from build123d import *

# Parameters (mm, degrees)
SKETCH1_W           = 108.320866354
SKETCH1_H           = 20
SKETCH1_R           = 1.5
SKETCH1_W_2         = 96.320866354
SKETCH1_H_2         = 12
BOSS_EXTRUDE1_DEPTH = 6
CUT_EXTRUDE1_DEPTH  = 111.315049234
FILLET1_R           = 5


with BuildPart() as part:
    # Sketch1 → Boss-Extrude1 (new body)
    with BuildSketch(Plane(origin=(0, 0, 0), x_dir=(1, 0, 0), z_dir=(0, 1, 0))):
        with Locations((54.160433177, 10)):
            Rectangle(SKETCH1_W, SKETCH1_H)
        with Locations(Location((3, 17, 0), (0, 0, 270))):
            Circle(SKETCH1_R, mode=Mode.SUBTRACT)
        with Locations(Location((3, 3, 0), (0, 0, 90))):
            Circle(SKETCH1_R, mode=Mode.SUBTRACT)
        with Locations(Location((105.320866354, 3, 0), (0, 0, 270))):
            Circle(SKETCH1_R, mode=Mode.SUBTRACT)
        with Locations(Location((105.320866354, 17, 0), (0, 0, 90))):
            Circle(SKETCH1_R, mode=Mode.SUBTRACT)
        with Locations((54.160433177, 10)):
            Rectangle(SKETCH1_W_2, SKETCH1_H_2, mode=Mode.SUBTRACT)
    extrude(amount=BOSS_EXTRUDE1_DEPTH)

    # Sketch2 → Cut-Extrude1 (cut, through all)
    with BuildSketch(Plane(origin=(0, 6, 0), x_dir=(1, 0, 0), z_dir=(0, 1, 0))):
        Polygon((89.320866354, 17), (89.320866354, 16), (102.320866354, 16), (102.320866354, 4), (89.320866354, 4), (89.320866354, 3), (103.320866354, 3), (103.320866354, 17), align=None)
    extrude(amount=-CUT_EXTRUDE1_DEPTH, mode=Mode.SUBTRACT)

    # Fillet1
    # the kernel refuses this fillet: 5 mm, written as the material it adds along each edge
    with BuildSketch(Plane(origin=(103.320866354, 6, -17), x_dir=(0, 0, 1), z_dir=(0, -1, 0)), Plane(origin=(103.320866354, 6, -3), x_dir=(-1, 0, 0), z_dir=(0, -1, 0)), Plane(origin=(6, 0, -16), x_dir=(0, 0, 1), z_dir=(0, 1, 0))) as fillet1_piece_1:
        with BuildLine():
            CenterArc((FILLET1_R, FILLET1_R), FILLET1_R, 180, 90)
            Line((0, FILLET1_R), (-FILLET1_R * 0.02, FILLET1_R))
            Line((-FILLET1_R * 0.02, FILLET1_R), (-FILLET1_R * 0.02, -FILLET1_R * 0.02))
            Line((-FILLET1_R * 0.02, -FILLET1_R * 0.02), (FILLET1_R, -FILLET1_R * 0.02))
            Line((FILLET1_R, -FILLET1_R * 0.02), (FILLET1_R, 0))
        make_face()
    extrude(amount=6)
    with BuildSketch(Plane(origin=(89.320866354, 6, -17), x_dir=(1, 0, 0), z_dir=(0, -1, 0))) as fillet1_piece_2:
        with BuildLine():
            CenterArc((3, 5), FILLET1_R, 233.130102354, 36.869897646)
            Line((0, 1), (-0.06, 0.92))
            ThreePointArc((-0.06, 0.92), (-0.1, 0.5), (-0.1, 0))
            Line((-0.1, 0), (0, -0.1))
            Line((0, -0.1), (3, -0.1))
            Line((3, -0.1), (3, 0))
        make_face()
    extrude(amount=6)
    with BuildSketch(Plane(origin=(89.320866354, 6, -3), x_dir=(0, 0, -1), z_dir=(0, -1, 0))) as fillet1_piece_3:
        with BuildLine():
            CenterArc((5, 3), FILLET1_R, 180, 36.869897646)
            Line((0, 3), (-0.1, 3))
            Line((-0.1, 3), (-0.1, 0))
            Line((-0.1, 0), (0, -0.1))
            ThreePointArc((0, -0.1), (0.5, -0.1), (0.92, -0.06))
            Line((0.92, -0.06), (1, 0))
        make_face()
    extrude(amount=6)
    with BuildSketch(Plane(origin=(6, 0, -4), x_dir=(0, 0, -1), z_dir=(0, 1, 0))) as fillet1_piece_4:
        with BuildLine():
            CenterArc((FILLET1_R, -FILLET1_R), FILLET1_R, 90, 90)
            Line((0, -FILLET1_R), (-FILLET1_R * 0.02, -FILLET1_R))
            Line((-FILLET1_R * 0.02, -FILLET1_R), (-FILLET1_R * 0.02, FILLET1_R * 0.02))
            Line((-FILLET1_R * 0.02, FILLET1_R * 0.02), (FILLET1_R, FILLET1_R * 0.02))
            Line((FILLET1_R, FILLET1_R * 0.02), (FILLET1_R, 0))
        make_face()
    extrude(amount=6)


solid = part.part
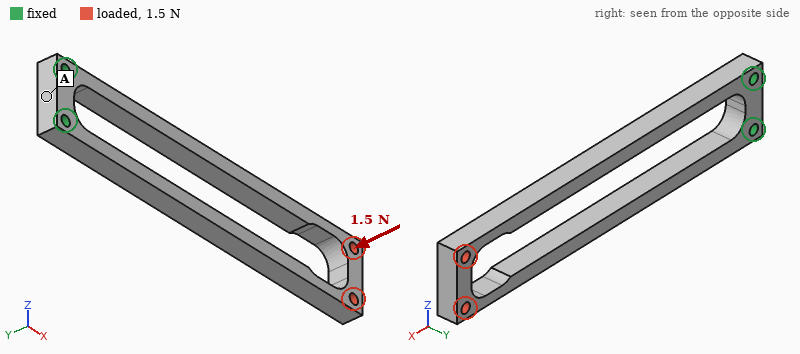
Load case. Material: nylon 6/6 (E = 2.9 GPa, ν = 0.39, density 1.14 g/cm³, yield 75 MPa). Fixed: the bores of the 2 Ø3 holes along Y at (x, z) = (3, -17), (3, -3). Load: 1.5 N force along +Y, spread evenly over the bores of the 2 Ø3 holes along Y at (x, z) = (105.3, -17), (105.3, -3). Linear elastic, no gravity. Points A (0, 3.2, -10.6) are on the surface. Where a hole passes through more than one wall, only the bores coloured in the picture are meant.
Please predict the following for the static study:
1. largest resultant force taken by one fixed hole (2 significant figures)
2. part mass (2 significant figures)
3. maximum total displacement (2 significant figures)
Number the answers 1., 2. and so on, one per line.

1. 0.75 N
2. 6.6 g
3. 1.3 mm
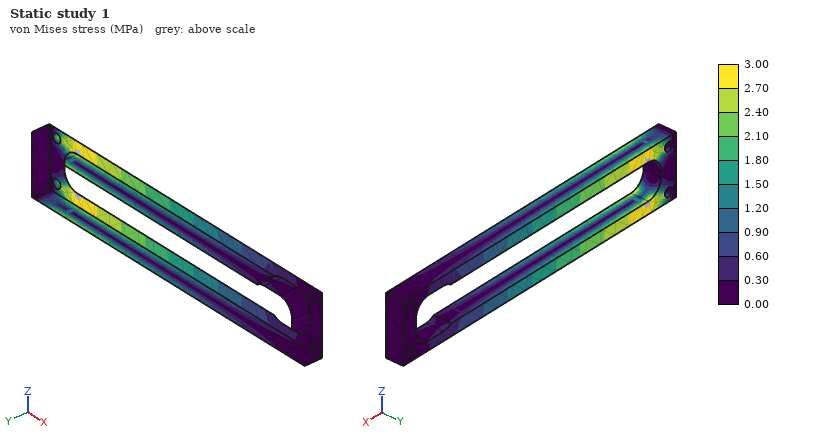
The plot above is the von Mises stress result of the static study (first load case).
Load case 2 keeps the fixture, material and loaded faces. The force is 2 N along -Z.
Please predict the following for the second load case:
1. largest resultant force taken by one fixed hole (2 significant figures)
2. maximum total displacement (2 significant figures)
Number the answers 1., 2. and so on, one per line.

1. 10 N
2. 1.2 mm
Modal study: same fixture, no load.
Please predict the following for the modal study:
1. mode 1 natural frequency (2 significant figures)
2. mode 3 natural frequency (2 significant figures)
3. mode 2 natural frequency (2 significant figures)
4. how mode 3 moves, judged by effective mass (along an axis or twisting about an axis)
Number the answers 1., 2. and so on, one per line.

1. 130 Hz
2. 520 Hz
3. 140 Hz
4. twisting about X
